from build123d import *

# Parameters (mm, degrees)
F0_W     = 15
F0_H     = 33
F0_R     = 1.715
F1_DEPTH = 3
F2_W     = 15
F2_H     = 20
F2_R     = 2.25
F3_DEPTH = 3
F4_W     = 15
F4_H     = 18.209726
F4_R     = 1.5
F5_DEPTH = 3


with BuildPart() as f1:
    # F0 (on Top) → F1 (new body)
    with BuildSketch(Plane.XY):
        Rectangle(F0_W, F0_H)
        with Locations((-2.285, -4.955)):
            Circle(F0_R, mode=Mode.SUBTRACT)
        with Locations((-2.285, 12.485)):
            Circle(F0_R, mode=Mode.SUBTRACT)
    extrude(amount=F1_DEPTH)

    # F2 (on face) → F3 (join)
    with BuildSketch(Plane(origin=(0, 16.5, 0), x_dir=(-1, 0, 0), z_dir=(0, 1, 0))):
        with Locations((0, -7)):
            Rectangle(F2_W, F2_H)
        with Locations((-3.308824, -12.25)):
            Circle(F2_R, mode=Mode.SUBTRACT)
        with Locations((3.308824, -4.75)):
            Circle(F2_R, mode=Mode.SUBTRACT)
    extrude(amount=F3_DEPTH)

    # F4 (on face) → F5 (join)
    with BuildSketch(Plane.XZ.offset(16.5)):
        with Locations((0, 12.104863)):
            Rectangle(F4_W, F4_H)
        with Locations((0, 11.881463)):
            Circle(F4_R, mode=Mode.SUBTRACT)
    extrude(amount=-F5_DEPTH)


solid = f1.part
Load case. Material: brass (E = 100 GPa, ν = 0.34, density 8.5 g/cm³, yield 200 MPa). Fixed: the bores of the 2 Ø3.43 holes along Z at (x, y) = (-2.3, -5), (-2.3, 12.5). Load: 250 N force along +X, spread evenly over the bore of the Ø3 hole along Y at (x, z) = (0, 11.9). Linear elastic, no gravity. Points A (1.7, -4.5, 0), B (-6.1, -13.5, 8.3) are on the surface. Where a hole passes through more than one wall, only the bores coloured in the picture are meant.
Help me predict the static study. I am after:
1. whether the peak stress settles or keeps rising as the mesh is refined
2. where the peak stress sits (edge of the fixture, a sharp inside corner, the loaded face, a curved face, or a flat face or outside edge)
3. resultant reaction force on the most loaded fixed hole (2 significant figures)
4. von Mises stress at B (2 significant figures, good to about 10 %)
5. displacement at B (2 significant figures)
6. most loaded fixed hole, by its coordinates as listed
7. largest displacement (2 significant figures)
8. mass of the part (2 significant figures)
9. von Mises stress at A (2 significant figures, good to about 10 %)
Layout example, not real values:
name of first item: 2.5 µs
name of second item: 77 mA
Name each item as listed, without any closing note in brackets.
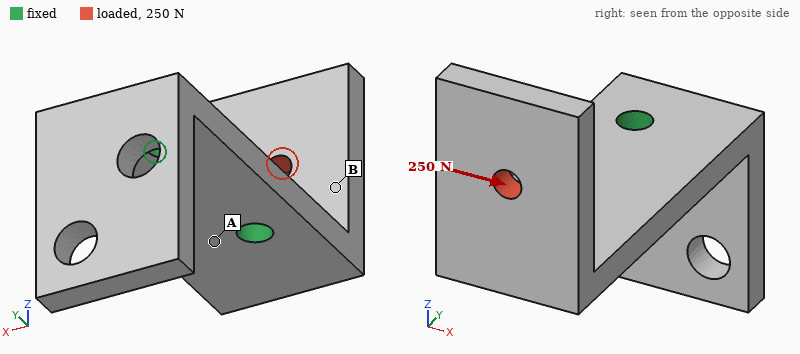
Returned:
whether the peak stress settles or keeps rising as the mesh is refined: keeps rising
where the peak stress sits: edge of the fixture
resultant reaction force on the most loaded fixed hole: 350 N
von Mises stress at B: 22 MPa
displacement at B: 0.040 mm
most loaded fixed hole, by its coordinates as listed: (-2.3, -5)
largest displacement: 0.10 mm
mass of the part: 26 g
von Mises stress at A: 65 MPa
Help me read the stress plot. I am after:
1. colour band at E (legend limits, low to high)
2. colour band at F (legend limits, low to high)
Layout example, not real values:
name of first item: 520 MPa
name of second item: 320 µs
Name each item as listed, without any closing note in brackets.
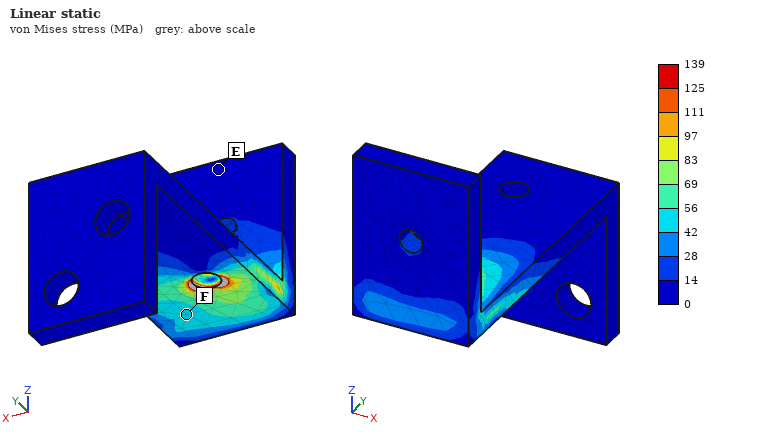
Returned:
colour band at E: 0 to 14 MPa
colour band at F: 42 to 56 MPa
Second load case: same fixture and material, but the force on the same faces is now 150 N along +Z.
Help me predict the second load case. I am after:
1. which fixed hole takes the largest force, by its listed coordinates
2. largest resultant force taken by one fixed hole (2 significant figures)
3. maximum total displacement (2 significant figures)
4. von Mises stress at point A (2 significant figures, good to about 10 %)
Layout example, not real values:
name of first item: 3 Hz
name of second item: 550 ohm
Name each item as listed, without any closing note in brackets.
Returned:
which fixed hole takes the largest force, by its listed coordinates: (-2.3, -5)
largest resultant force taken by one fixed hole: 170 N
maximum total displacement: 48 µm
von Mises stress at point A: 27 MPa
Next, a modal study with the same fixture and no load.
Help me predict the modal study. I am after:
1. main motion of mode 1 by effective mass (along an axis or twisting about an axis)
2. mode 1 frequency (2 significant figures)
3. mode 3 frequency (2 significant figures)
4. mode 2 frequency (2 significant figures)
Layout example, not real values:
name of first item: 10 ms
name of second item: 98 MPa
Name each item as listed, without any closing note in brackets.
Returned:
main motion of mode 1 by effective mass: along Y
mode 1 frequency: 2400 Hz
mode 3 frequency: 3500 Hz
mode 2 frequency: 3500 Hz
